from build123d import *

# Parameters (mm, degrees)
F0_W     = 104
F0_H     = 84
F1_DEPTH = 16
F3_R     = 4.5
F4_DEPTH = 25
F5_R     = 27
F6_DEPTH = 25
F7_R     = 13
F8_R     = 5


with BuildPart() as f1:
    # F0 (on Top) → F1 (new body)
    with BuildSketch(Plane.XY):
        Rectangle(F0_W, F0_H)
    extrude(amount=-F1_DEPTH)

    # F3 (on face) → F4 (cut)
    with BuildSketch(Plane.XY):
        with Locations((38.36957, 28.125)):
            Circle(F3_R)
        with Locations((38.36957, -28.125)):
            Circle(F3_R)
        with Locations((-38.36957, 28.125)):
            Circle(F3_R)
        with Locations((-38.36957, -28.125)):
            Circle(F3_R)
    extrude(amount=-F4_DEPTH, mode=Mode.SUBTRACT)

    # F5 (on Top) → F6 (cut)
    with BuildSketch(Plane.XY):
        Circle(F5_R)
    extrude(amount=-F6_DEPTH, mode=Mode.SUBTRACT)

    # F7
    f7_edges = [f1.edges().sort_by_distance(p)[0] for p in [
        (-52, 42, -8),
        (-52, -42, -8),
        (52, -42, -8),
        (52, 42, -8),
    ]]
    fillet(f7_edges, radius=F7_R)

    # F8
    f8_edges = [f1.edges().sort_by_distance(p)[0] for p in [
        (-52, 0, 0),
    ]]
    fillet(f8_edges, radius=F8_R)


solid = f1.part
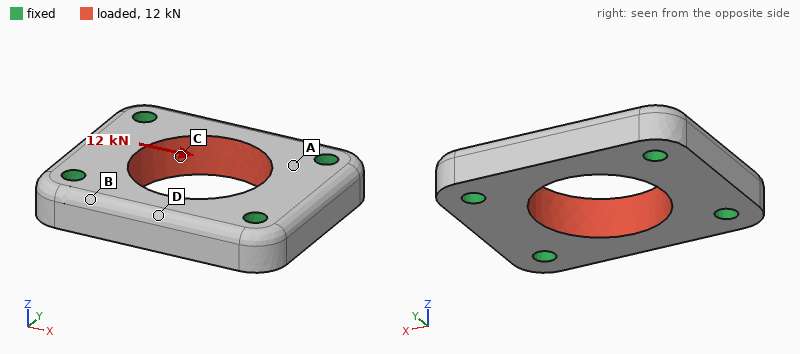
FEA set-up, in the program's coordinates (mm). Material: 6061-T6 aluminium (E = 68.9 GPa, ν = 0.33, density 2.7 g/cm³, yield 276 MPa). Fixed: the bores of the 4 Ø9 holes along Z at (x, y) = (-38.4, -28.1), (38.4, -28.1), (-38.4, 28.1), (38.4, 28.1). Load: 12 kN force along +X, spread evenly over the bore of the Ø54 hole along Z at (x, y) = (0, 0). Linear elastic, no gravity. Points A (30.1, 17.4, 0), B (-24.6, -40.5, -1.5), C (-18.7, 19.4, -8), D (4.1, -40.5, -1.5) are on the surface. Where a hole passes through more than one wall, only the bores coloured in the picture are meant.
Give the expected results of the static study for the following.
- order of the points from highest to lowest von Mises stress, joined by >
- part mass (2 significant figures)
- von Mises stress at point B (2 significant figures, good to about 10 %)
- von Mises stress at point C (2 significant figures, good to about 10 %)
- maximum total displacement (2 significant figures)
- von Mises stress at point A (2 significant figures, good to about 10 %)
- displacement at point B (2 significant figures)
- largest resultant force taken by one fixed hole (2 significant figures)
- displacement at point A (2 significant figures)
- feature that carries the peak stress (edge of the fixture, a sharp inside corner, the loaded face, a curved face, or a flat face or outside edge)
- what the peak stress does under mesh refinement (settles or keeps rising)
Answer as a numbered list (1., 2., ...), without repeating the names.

1. C > A > B > D
2. 260 g
3. 3.3 MPa
4. 7.7 MPa
5. 4.1 µm
6. 5.7 MPa
7. 0.83 µm
8. 3.0 kN
9. 1.9 µm
10. edge of the fixture
11. keeps rising
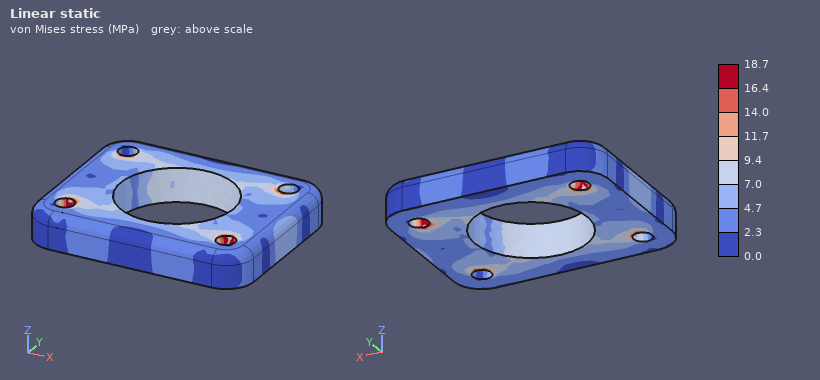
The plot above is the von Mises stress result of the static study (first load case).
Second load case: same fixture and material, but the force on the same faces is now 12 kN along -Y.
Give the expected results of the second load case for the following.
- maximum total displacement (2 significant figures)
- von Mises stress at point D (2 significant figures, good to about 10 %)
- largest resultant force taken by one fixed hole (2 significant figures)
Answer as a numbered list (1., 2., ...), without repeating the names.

1. 11 µm
2. 14 MPa
3. 3.0 kN
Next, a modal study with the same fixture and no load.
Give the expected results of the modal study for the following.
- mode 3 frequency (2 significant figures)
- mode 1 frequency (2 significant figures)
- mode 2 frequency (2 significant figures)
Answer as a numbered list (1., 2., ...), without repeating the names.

1. 15 kHz
2. 13 kHz
3. 13 kHz
